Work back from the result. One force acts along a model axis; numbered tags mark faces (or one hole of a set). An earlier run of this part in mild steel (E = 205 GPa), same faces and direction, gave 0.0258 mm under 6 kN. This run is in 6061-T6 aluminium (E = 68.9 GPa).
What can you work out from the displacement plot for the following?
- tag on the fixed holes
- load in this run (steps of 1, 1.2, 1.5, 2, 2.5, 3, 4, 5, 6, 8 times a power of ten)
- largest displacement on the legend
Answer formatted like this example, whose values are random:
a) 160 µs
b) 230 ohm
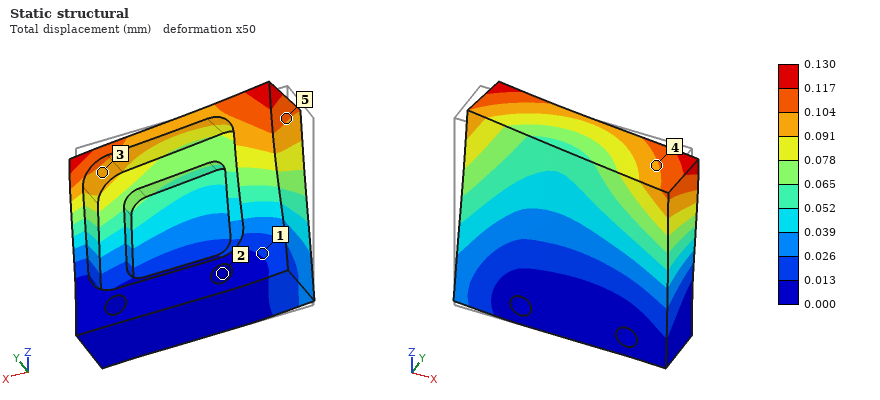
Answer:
a) 2
b) 10 kN
c) 0.130 mm
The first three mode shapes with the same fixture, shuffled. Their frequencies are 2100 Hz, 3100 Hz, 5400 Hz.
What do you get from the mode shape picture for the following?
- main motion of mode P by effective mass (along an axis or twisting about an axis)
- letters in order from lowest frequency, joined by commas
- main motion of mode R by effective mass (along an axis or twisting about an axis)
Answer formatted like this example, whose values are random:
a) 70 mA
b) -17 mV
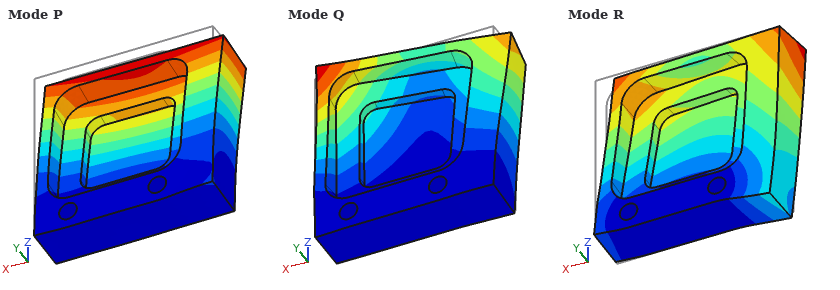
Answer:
a) along Y
b) P, Q, R
c) along X
